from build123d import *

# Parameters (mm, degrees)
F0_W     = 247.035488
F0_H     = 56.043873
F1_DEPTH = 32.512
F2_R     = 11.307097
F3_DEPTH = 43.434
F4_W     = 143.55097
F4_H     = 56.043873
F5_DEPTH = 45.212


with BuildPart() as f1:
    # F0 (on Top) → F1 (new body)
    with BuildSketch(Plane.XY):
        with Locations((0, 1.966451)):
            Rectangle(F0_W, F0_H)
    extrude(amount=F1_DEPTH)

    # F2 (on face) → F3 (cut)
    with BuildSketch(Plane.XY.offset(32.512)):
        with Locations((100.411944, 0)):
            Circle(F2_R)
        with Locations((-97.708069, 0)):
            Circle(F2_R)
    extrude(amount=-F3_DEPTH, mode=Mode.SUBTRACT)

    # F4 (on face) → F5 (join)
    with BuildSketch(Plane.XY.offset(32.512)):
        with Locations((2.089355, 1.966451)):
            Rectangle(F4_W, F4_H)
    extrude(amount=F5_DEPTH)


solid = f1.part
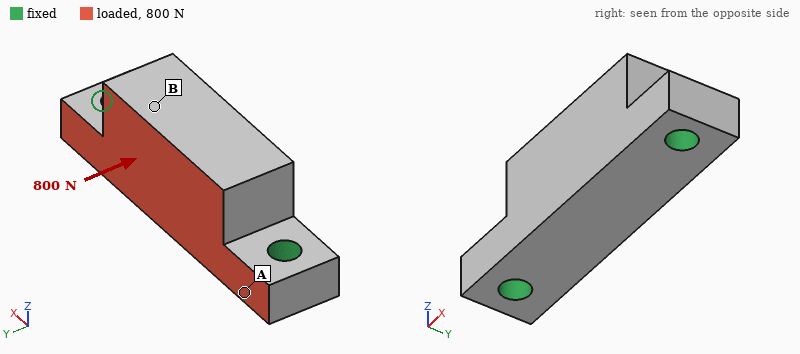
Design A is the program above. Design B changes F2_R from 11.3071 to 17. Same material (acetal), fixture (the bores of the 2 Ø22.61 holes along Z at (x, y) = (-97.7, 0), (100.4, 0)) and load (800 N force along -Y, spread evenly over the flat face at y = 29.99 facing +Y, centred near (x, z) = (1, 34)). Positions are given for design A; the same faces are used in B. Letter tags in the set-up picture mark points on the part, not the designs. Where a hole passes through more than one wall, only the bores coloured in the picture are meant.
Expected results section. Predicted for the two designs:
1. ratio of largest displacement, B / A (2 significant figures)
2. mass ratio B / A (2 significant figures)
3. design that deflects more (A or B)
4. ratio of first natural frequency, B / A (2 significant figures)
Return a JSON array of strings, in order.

["0.74", "0.96", "A", "1.2"]
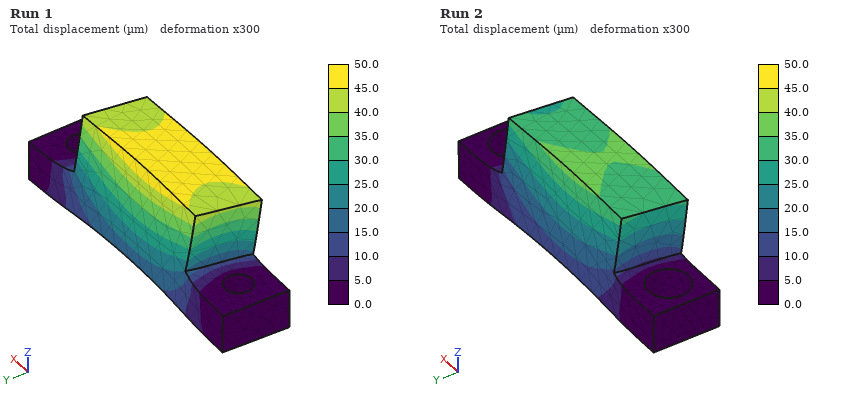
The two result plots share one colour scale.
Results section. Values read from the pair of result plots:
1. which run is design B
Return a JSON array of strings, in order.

["Run 2"]
